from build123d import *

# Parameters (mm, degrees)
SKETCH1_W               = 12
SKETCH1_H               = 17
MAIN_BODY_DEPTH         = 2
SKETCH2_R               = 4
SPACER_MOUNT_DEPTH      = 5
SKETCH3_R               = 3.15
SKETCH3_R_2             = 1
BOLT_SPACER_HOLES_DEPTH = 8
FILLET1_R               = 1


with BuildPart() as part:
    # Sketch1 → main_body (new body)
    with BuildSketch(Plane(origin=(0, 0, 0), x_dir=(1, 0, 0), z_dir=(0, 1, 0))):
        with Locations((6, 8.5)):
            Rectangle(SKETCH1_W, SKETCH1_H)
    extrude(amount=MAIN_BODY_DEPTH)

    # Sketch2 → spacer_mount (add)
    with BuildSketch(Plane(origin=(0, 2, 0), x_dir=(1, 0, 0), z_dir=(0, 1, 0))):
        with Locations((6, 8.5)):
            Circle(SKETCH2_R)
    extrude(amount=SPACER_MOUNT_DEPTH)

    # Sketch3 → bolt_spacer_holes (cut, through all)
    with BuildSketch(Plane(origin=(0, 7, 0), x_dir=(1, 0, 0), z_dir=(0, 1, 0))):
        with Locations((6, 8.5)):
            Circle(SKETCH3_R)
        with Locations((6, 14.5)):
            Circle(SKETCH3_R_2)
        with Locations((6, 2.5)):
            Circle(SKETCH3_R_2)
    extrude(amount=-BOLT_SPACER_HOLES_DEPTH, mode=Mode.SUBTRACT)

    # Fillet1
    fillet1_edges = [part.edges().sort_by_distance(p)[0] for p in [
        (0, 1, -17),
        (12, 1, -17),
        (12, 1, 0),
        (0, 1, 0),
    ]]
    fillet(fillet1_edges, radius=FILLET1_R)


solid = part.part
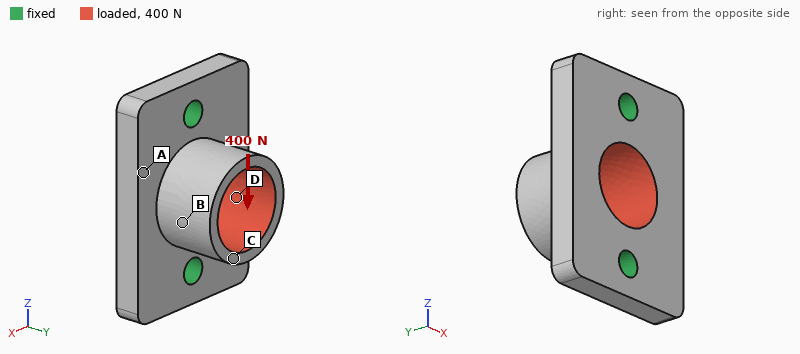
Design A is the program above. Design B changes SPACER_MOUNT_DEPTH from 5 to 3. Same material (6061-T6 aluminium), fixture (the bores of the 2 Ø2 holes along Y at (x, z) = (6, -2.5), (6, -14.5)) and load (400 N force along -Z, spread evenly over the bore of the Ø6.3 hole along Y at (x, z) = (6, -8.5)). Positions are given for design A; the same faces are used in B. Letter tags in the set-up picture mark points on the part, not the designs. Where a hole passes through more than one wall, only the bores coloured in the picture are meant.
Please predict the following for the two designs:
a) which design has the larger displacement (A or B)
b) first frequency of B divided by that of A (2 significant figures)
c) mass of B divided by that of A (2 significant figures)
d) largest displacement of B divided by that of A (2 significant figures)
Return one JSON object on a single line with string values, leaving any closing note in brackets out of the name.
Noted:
{"which design has the larger displacement": "A", "first frequency of B divided by that of A": "1.2", "mass of B divided by that of A": "0.91", "largest displacement of B divided by that of A": "0.59"}
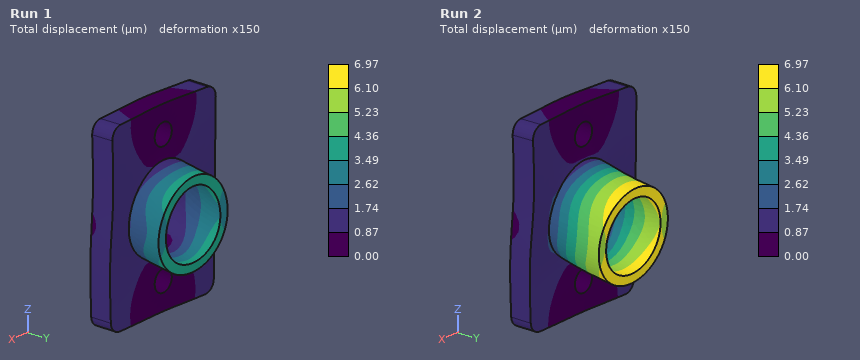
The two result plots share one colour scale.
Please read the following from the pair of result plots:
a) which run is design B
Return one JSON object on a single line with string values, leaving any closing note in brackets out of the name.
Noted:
{"which run is design B": "Run 1"}
